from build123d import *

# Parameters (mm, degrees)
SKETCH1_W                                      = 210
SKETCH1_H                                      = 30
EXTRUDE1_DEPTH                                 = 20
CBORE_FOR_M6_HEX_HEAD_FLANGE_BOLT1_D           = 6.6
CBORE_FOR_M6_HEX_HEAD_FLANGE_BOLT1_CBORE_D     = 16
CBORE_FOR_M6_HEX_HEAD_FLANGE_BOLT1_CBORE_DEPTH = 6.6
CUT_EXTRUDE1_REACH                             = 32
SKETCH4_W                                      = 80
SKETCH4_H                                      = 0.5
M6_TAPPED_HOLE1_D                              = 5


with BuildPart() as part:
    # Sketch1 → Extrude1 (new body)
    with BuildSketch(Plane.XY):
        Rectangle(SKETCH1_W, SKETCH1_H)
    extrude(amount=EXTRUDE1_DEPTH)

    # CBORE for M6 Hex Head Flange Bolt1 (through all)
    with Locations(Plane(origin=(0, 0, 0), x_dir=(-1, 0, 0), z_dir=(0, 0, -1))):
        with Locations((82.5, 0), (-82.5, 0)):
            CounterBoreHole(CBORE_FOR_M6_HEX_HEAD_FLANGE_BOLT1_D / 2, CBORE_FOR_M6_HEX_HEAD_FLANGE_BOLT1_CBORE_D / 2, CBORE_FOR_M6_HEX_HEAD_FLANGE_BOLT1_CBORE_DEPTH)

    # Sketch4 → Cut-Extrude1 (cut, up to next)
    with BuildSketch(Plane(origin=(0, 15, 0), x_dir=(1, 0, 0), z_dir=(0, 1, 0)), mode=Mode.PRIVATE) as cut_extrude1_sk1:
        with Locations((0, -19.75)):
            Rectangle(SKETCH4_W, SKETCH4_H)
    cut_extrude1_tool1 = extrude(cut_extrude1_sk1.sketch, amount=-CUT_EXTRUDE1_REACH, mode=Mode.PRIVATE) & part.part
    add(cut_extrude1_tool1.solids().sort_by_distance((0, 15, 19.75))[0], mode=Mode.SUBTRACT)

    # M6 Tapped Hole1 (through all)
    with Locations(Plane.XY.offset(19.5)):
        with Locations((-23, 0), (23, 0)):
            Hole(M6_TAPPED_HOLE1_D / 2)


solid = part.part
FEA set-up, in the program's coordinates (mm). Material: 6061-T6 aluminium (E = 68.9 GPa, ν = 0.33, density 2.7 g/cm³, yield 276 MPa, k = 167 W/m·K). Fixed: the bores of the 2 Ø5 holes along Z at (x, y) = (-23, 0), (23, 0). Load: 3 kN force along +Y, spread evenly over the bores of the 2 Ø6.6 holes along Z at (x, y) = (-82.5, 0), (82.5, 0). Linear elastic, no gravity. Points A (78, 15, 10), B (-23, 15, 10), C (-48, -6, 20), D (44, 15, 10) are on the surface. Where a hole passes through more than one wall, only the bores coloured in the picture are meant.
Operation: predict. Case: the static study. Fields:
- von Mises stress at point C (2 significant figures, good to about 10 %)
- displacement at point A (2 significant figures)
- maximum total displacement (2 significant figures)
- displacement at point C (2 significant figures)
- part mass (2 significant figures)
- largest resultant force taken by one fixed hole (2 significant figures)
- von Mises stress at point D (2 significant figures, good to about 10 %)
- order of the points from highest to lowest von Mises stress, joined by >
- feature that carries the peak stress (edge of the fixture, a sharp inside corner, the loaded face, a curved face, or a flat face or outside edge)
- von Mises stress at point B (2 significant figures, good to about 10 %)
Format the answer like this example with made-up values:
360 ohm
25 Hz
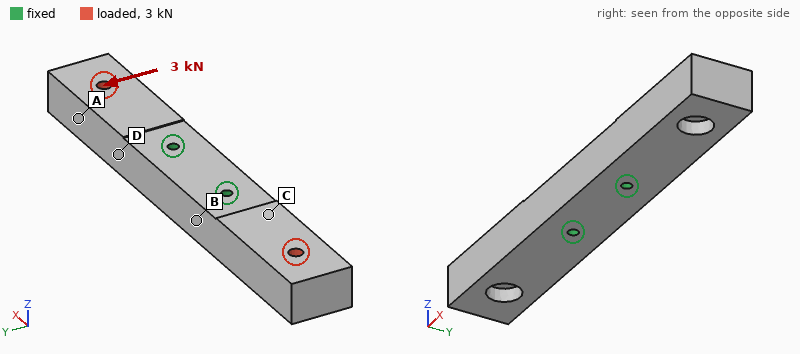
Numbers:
11 MPa
0.069 mm
0.11 mm
0.026 mm
330 g
1.5 kN
20 MPa
B > D > C > A
edge of the fixture
27 MPa
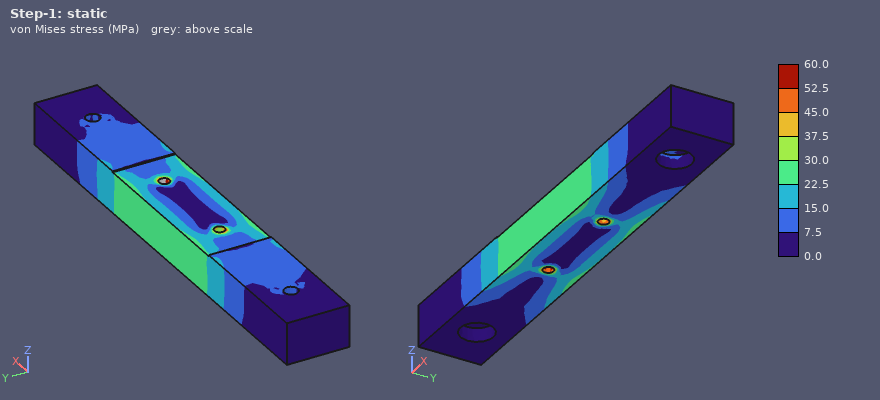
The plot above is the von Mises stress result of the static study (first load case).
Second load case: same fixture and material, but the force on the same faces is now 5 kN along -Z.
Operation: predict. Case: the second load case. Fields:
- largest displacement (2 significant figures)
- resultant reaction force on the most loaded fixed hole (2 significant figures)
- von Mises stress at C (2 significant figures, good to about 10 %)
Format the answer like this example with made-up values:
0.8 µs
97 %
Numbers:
0.26 mm
2.5 kN
41 MPa
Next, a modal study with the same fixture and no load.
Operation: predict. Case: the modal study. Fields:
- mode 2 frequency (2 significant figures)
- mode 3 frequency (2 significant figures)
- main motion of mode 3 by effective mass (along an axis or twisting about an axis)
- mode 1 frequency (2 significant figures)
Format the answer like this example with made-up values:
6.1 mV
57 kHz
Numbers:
2200 Hz
2600 Hz
along Y
2200 Hz
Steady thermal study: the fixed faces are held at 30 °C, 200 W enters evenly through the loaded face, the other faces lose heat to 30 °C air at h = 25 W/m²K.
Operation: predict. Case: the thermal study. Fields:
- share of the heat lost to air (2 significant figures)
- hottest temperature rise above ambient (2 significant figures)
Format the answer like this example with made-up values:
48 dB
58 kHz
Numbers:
9.3 %
68 K
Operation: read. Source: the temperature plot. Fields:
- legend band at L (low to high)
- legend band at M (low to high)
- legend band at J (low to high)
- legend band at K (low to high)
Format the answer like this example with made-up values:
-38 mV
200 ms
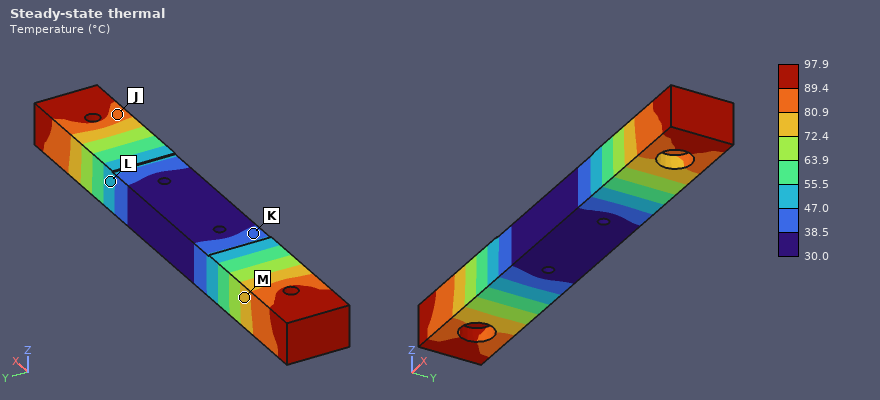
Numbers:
47.0 to 55.5 °C
72.4 to 80.9 °C
80.9 to 89.4 °C
38.5 to 47.0 °C
